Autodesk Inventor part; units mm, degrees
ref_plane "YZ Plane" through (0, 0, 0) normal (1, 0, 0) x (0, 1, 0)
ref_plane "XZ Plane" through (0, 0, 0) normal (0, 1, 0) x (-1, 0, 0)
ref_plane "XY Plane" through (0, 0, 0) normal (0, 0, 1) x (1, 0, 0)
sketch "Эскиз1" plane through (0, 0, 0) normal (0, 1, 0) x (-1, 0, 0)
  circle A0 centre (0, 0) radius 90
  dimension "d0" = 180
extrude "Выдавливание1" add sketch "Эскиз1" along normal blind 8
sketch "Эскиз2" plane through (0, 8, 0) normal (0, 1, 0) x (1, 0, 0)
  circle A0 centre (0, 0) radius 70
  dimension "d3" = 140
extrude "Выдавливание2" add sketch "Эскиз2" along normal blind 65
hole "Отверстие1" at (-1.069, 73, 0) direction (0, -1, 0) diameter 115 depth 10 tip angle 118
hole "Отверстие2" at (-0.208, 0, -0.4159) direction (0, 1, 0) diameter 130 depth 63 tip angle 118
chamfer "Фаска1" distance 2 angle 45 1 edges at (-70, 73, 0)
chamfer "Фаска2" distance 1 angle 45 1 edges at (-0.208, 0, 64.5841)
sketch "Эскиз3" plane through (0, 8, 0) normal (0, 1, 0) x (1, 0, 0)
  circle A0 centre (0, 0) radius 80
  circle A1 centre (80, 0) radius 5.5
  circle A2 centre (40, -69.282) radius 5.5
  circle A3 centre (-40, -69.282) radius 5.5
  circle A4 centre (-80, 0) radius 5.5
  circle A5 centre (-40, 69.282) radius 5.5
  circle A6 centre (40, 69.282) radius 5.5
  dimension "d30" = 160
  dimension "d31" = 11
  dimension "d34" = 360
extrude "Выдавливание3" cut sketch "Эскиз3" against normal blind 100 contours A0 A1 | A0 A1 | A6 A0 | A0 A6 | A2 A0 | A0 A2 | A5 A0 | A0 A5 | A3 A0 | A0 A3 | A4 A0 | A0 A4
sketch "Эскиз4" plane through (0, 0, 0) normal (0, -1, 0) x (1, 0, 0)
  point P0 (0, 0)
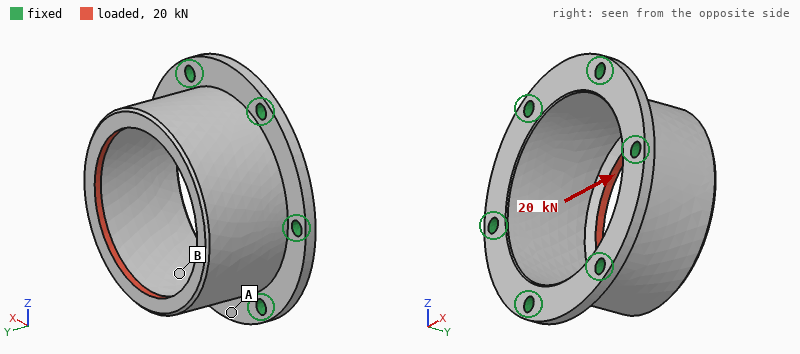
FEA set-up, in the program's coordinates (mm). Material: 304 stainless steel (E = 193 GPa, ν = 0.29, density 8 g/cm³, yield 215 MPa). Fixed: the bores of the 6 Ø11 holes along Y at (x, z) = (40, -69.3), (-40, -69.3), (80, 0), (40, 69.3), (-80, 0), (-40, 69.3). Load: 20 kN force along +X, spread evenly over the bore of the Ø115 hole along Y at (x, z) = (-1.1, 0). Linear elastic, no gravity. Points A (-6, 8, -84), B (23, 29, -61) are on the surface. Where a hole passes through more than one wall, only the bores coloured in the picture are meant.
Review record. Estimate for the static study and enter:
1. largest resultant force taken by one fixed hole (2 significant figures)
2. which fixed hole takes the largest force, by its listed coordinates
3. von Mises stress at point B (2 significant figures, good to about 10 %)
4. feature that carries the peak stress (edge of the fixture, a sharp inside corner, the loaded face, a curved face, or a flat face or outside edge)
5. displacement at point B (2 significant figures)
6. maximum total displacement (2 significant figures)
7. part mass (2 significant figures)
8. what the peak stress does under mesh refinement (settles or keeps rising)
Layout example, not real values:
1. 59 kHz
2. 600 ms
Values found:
1. 7.0 kN
2. (-80, 0)
3. 35 MPa
4. edge of the fixture
5. 9.6 µm
6. 53 µm
7. 2.0 kg
8. keeps rising
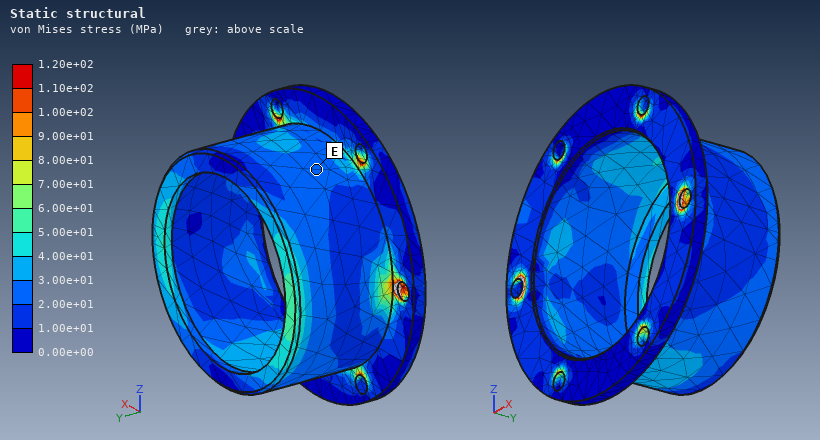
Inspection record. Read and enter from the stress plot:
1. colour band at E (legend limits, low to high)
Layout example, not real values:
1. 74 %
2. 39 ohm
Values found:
1. 2.00e+01 to 3.00e+01 MPa
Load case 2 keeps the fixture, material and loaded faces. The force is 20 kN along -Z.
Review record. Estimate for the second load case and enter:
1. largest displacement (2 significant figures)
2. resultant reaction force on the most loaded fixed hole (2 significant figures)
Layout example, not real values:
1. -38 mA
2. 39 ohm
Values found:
1. 48 µm
2. 6.6 kN
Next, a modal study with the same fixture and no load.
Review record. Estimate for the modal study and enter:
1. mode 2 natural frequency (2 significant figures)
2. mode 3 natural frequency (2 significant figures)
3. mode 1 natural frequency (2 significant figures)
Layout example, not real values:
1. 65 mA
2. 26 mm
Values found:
1. 2900 Hz
2. 4400 Hz
3. 2900 Hz
